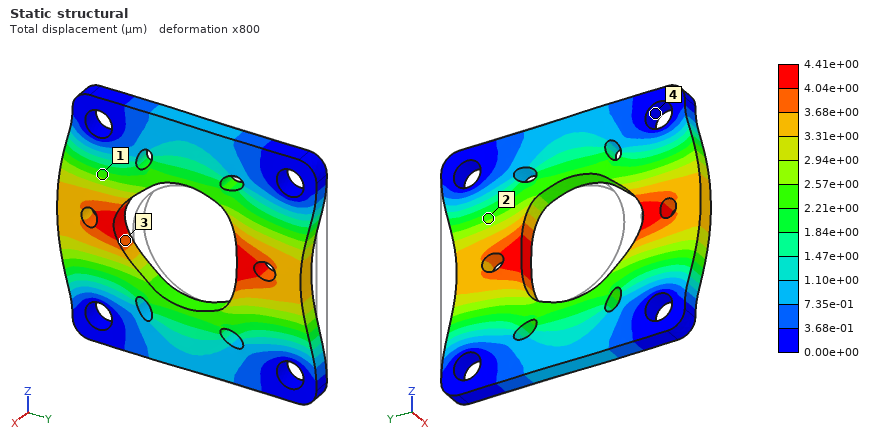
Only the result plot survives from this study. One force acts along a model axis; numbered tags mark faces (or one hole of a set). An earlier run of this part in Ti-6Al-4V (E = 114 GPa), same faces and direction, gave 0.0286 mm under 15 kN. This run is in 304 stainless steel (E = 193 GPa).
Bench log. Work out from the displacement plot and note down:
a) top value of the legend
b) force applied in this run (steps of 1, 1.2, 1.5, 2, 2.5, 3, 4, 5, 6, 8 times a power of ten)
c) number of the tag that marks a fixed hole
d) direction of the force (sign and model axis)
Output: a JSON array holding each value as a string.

["4.41e+00 µm", "4 kN", "4", "-Y"]
